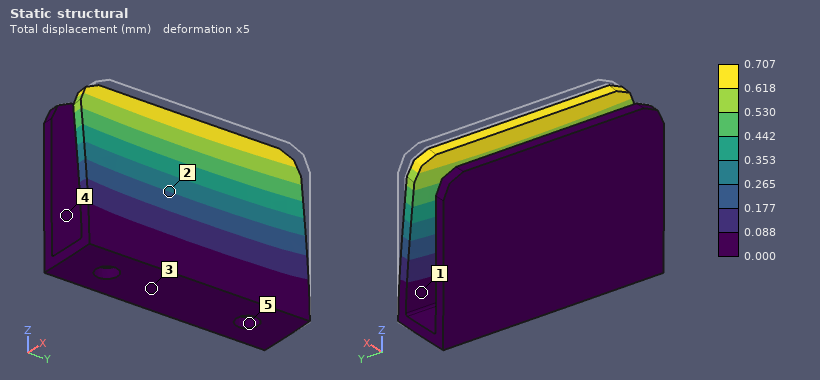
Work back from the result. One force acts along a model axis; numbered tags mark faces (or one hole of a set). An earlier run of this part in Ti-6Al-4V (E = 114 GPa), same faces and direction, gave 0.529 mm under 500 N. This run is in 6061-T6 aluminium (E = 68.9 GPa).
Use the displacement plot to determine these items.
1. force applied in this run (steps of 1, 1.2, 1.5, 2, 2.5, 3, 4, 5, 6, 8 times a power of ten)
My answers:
400 N
